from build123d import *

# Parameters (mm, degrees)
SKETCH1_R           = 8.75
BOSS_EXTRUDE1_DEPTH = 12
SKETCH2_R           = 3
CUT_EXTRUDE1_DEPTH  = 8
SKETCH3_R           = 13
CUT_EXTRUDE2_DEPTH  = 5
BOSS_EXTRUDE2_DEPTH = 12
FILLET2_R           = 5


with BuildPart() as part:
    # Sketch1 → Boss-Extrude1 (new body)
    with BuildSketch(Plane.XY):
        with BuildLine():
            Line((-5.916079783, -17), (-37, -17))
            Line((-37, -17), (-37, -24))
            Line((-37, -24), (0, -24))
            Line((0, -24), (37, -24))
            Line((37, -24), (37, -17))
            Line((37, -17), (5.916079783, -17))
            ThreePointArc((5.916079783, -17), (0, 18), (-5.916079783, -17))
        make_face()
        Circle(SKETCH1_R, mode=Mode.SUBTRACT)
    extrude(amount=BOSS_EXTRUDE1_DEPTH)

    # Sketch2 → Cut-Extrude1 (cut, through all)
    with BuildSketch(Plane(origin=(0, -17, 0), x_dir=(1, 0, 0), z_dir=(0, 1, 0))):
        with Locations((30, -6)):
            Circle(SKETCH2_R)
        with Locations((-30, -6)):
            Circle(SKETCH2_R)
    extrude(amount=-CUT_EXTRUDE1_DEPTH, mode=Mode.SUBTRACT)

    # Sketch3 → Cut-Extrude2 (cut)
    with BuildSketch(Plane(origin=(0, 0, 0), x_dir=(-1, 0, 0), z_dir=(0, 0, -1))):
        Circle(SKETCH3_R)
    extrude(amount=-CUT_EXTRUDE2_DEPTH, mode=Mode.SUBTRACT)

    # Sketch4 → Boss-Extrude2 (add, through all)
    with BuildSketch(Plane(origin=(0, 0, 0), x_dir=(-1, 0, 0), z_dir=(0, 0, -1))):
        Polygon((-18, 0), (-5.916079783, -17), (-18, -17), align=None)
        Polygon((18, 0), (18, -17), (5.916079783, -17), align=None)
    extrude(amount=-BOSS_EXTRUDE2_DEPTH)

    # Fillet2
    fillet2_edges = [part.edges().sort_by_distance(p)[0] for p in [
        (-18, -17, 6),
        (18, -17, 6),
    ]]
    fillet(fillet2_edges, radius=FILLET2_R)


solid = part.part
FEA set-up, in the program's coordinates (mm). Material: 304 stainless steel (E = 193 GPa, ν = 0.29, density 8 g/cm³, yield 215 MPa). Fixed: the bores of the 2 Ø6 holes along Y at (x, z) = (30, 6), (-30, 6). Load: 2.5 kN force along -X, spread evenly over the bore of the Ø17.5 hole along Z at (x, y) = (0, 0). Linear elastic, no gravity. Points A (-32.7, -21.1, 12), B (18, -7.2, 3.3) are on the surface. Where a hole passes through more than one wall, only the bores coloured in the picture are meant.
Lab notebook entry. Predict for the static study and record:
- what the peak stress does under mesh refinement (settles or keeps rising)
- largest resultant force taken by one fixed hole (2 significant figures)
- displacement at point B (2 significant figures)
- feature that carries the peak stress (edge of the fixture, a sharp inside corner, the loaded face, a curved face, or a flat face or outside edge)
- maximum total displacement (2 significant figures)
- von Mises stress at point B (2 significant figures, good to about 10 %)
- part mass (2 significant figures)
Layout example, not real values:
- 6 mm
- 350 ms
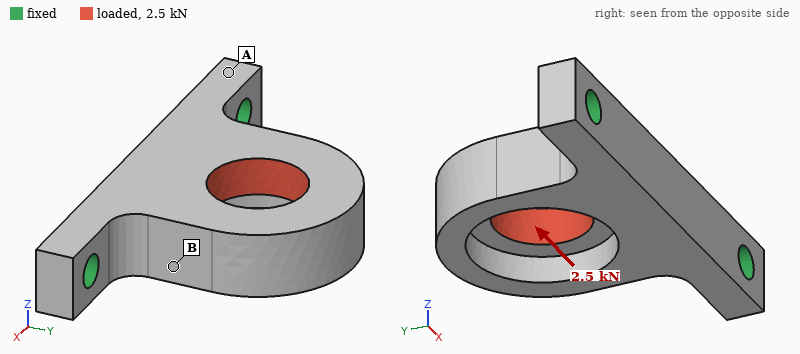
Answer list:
- keeps rising
- 1.6 kN
- 5.8 µm
- edge of the fixture
- 14 µm
- 25 MPa
- 120 g
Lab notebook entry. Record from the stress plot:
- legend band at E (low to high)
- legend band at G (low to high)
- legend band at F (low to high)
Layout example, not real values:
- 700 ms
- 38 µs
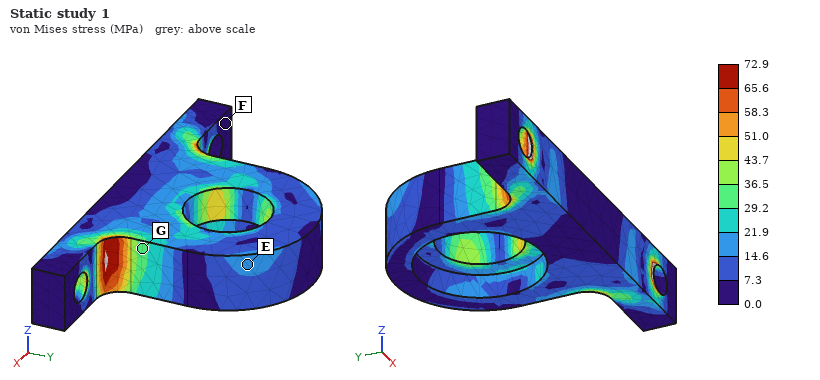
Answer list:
- 14.6 to 21.9 MPa
- 29.2 to 36.5 MPa
- 0.0 to 7.3 MPa
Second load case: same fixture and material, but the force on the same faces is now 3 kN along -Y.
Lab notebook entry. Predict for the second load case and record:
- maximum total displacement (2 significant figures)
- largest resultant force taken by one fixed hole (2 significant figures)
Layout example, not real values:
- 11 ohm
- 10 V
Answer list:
- 30 µm
- 1.8 kN
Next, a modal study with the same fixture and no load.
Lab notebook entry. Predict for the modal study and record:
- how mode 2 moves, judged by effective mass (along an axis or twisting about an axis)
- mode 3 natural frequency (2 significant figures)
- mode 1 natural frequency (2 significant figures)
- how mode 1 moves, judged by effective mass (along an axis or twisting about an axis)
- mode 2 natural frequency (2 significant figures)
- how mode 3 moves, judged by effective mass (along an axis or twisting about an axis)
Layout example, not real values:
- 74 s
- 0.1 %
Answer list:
- along X
- 9800 Hz
- 2800 Hz
- along Z
- 8900 Hz
- along Y
